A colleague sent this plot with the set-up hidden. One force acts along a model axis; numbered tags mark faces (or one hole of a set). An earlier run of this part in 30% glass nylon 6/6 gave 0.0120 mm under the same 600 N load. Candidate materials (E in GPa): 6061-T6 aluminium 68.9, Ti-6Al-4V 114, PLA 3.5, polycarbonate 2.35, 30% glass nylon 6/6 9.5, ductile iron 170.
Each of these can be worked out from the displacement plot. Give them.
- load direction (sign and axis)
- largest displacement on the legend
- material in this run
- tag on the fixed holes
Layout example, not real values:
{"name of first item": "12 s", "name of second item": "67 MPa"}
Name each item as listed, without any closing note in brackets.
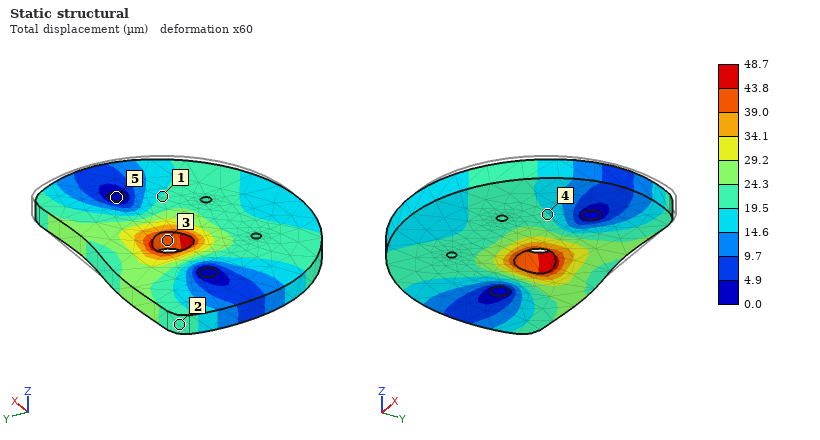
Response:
{"load direction": "-X", "largest displacement on the legend": "48.7 µm", "material in this run": "polycarbonate", "tag on the fixed holes": "5"}
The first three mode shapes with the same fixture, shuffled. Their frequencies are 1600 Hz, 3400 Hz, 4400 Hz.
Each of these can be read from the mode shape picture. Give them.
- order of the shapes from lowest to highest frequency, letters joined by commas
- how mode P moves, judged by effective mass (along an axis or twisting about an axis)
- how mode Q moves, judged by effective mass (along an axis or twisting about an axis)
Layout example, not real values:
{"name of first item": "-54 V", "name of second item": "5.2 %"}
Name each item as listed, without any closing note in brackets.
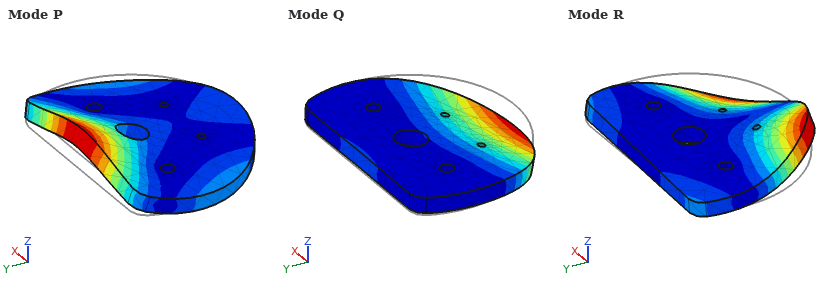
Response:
{"order of the shapes from lowest to highest frequency, letters joined by commas": "Q, R, P", "how mode P moves, judged by effective mass": "along Z", "how mode Q moves, judged by effective mass": "along Z"}
